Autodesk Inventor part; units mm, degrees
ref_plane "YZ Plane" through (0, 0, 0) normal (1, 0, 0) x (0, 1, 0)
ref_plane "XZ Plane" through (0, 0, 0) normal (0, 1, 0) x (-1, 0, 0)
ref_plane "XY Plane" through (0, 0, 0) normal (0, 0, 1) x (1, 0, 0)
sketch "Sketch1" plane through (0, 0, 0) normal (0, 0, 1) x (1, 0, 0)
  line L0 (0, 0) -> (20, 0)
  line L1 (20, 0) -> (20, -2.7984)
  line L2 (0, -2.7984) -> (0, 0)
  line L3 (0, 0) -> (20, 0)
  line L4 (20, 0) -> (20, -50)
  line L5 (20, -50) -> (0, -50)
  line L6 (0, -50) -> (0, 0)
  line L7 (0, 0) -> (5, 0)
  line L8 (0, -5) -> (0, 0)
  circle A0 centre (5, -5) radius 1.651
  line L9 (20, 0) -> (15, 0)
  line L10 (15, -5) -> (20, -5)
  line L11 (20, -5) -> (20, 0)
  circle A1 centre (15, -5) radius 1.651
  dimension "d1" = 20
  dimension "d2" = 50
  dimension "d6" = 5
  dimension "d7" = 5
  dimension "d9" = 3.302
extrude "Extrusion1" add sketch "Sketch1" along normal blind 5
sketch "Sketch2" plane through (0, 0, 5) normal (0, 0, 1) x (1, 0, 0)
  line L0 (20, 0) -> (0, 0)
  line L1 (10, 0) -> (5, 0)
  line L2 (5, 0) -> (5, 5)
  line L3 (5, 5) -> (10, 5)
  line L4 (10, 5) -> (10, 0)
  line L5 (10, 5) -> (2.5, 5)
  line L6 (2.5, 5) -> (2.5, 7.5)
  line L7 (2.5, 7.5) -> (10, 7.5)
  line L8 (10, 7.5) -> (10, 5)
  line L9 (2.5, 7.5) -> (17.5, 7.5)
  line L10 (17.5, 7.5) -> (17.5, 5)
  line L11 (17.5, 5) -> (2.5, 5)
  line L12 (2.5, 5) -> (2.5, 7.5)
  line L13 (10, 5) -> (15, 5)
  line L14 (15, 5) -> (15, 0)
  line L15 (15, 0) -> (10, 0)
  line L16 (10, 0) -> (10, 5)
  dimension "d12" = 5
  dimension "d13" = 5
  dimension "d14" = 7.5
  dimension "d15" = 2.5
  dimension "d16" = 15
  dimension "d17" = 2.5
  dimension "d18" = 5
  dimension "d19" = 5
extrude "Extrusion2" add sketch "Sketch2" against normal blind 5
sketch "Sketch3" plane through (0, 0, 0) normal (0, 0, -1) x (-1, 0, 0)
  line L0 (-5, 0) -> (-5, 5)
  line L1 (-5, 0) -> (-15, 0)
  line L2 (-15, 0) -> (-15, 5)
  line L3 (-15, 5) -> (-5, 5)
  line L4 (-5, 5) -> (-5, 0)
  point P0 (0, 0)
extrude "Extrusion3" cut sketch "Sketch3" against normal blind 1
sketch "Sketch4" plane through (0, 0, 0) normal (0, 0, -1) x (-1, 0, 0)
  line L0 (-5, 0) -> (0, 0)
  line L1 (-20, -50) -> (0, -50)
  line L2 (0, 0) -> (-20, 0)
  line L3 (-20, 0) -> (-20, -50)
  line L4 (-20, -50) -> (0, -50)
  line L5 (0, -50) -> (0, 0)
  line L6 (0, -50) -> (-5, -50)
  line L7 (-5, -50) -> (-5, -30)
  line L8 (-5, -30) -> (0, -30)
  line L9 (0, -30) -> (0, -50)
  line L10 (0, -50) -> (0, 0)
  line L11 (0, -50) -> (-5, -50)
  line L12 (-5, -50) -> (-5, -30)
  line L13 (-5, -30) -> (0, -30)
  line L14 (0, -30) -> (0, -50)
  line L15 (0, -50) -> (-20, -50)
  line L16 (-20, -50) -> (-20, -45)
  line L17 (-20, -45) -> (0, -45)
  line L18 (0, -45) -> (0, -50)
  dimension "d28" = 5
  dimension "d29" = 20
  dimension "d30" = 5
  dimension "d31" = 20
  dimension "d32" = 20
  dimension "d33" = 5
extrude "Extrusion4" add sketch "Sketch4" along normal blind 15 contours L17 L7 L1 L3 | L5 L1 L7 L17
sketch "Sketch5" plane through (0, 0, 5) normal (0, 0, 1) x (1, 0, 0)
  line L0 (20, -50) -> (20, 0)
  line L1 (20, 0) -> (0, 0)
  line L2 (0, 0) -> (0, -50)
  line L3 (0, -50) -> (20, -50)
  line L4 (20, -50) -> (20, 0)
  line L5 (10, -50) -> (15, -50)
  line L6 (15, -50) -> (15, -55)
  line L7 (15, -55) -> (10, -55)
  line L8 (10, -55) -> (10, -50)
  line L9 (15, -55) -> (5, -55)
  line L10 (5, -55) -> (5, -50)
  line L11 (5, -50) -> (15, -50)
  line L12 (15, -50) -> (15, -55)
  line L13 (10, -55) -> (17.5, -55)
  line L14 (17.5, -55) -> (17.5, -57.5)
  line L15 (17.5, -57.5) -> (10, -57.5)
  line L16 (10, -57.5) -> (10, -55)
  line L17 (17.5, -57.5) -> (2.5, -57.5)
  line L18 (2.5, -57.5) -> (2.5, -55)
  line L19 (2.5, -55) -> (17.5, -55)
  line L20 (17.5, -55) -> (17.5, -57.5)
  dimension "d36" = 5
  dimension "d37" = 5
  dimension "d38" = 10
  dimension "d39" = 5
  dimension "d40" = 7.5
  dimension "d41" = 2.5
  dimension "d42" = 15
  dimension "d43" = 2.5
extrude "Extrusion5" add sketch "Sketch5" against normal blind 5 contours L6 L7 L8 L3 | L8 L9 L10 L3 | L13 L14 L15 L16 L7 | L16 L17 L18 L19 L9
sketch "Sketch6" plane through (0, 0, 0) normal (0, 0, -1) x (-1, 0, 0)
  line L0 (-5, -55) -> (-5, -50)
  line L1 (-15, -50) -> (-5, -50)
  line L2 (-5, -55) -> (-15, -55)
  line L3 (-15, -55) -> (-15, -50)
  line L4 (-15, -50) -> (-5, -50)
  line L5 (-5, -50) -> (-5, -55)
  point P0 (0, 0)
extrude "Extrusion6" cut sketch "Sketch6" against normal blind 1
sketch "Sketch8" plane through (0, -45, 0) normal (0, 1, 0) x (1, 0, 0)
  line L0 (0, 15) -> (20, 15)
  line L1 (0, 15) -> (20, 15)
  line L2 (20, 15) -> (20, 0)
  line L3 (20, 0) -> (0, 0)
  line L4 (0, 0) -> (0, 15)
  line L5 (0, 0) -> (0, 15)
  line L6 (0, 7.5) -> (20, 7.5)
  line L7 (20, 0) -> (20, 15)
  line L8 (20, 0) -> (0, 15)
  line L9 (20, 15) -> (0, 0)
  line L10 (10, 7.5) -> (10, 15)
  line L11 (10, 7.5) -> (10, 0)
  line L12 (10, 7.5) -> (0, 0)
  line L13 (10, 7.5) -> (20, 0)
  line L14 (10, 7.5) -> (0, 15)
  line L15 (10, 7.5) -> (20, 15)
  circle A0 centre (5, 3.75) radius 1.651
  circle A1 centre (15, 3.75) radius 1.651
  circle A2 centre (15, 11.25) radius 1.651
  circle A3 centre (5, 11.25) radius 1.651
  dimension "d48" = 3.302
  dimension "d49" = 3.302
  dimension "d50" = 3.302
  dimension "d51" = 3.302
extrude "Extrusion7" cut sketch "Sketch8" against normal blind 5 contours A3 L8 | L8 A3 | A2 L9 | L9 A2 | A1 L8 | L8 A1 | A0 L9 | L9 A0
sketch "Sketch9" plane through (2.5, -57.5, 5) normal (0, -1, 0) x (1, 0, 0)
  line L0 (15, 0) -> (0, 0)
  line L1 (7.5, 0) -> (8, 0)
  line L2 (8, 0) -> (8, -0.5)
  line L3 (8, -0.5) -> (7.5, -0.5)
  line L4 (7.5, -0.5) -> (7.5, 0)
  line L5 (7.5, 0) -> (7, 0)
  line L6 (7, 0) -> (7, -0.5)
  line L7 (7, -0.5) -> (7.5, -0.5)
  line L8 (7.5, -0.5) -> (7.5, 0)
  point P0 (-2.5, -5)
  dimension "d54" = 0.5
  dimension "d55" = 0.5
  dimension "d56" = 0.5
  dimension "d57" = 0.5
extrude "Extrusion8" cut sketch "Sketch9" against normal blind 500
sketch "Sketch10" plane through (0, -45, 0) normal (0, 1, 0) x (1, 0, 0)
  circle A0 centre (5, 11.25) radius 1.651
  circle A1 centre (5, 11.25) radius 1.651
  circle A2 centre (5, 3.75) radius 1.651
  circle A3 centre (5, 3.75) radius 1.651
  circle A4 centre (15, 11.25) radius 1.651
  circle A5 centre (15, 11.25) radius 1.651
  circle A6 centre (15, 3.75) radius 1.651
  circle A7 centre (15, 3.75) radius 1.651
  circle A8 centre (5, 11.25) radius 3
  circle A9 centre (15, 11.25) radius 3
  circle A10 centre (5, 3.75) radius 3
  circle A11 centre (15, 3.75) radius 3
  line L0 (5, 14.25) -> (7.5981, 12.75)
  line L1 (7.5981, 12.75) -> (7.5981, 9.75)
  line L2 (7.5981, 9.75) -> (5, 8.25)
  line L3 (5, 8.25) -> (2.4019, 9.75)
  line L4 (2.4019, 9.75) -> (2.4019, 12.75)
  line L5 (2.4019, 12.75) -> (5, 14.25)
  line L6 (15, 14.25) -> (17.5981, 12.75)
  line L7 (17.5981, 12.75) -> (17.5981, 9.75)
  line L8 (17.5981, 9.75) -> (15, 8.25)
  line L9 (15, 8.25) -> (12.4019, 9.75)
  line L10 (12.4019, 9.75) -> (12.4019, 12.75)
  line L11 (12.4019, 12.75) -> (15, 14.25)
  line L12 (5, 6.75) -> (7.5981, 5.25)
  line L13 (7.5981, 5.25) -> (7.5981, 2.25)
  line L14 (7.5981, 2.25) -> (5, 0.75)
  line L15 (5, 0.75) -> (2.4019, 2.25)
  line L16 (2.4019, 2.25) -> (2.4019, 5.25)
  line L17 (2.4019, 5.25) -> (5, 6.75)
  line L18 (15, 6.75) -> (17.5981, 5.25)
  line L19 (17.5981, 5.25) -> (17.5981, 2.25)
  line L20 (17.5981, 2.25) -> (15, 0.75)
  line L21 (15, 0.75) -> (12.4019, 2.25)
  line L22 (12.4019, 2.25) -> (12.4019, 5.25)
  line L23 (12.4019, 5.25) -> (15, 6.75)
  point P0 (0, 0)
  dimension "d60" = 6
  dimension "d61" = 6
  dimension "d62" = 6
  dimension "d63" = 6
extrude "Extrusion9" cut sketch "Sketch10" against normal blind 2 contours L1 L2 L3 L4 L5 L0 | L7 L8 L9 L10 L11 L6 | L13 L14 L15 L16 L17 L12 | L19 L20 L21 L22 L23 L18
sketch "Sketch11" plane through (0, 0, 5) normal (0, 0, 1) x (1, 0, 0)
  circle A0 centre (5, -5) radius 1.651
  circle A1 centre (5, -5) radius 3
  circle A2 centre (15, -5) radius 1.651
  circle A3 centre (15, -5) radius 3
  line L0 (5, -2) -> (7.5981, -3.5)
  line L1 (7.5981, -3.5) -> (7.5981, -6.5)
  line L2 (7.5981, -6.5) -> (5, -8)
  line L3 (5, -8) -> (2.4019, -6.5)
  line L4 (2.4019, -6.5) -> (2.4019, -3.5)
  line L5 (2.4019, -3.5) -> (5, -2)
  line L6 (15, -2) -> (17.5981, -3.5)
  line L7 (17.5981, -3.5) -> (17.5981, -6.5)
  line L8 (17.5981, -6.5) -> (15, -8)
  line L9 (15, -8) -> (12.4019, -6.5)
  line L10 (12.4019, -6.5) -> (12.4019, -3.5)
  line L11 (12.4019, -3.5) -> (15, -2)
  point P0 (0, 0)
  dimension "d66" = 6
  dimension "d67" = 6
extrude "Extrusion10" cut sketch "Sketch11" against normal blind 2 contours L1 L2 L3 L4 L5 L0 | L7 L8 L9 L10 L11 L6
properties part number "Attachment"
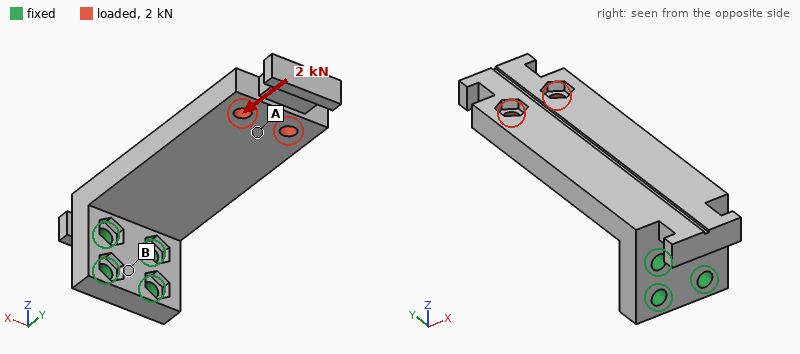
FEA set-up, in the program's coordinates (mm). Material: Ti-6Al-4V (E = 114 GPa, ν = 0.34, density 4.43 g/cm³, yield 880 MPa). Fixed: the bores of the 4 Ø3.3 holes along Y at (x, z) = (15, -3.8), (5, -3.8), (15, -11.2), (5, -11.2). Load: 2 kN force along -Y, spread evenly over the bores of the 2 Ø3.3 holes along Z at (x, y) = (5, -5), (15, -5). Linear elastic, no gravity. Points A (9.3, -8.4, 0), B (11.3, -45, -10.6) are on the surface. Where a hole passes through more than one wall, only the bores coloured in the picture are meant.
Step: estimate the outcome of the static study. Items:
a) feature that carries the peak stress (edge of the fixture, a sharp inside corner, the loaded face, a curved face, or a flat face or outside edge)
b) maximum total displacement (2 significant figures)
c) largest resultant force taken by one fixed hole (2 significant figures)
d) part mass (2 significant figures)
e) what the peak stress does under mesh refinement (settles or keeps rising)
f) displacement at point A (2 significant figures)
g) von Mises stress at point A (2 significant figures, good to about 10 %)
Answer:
edge of the fixture
36 µm
1.3 kN
30 g
keeps rising
32 µm
40 MPa
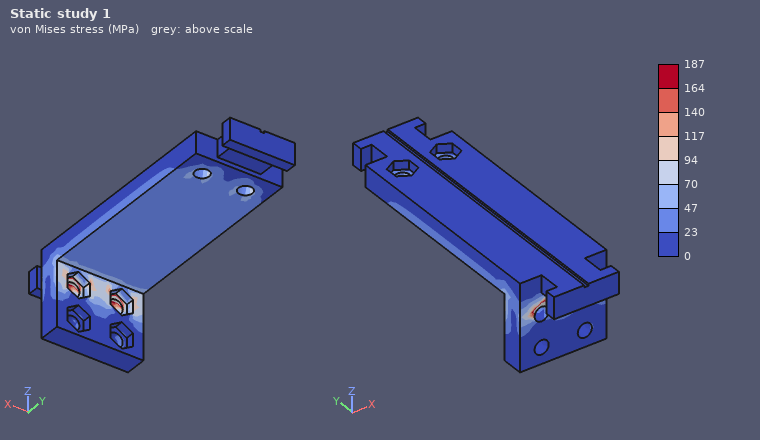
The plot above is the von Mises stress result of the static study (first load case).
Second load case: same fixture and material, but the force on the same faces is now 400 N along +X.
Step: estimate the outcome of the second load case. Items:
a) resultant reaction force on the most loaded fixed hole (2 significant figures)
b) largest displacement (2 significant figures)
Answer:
1.5 kN
0.13 mm
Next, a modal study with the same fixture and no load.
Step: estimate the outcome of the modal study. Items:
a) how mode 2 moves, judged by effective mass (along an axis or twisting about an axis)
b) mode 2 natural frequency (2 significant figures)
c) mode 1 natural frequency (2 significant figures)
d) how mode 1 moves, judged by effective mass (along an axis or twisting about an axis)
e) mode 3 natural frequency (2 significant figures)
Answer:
along X
3200 Hz
1300 Hz
along Z
7100 Hz
